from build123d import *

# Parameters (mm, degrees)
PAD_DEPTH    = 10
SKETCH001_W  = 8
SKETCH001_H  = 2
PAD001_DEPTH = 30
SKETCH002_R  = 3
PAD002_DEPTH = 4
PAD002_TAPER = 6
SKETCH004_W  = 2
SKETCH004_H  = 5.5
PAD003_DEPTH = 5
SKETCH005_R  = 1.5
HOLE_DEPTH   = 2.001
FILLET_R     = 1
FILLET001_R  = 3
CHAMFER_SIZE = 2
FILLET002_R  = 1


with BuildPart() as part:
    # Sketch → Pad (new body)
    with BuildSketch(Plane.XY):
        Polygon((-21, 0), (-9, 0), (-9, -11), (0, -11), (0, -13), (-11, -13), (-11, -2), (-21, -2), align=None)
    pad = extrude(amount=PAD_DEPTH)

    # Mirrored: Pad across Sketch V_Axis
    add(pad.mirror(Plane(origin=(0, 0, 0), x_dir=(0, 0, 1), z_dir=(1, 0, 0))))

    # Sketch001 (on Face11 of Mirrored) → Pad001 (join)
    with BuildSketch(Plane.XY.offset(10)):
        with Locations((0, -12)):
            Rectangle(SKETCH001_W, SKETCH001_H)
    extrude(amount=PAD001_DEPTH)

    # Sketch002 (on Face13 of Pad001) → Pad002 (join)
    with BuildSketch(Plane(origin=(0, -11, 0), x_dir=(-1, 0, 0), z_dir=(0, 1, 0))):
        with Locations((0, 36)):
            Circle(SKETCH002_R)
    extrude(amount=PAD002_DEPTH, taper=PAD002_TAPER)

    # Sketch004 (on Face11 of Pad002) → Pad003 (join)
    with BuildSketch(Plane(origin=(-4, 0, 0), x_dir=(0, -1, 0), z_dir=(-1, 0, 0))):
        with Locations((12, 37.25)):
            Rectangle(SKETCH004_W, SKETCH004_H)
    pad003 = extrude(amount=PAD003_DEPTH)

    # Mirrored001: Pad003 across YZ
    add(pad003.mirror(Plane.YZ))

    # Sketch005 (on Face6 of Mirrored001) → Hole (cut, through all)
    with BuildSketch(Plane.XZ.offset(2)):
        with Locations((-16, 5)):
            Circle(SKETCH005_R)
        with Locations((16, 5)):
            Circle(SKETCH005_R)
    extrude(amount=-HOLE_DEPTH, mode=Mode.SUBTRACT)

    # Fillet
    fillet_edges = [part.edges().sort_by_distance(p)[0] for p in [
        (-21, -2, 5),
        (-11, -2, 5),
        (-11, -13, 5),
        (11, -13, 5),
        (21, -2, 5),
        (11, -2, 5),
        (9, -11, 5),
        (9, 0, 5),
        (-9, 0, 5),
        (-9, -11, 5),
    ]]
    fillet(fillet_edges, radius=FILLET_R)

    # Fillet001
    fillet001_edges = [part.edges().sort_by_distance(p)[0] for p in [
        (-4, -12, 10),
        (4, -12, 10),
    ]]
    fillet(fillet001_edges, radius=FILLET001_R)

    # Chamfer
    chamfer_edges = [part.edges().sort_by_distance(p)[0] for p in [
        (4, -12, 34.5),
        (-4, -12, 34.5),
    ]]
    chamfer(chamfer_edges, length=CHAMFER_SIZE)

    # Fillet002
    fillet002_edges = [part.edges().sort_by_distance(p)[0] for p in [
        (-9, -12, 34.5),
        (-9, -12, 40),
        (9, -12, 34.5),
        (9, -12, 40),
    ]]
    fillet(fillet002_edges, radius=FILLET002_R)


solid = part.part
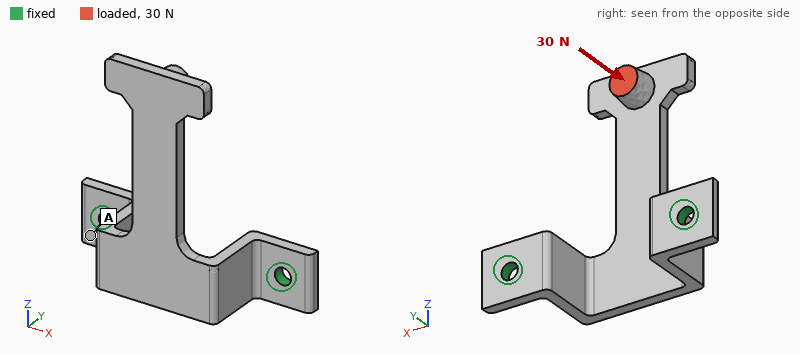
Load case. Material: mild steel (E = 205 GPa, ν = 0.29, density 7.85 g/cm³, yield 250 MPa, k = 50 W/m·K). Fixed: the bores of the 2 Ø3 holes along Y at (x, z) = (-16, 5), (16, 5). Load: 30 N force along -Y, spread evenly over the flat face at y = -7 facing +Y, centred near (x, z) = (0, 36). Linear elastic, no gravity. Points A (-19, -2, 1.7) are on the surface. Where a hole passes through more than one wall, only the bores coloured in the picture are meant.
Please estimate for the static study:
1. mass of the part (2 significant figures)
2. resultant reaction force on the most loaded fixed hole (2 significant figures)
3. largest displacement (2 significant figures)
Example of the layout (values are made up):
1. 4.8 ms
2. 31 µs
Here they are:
1. 15 g
2. 20 N
3. 0.31 mm
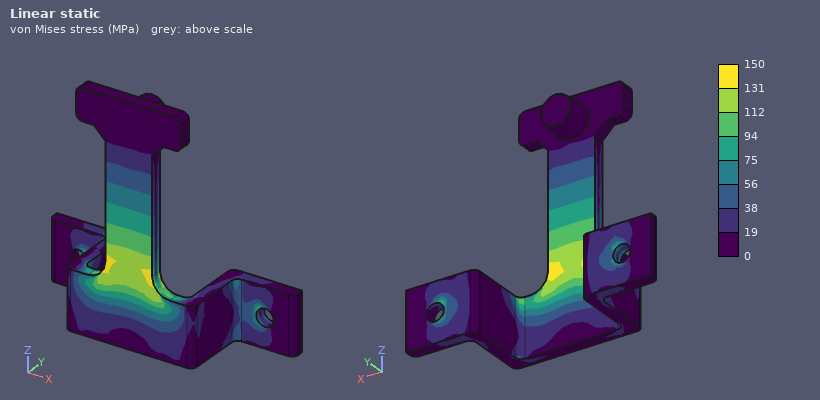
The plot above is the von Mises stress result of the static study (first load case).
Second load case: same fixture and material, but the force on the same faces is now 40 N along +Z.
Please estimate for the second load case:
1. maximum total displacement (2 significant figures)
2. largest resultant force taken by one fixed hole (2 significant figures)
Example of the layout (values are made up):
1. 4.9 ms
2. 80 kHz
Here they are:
1. 90 µm
2. 20 N
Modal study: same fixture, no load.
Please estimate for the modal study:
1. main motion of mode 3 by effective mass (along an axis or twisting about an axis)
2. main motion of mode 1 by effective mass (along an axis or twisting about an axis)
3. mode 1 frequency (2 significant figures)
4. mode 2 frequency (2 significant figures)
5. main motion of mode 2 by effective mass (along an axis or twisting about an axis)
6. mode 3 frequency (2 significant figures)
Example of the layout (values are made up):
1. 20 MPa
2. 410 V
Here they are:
1. along Z
2. along Y
3. 940 Hz
4. 2500 Hz
5. along X
6. 4500 Hz
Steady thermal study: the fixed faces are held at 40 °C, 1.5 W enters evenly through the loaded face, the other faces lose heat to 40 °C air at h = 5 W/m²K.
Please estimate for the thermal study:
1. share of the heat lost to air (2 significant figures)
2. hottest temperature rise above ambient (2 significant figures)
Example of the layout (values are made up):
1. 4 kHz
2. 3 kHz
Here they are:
1. 15 %
2. 63 K
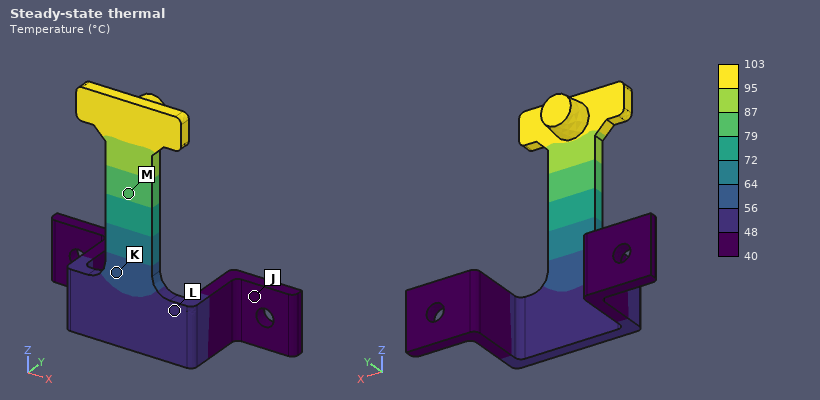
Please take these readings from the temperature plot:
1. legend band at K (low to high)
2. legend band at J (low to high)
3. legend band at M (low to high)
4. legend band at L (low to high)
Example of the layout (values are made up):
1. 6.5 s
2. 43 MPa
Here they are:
1. 56 to 64 °C
2. 40 to 48 °C
3. 79 to 87 °C
4. 48 to 56 °C
